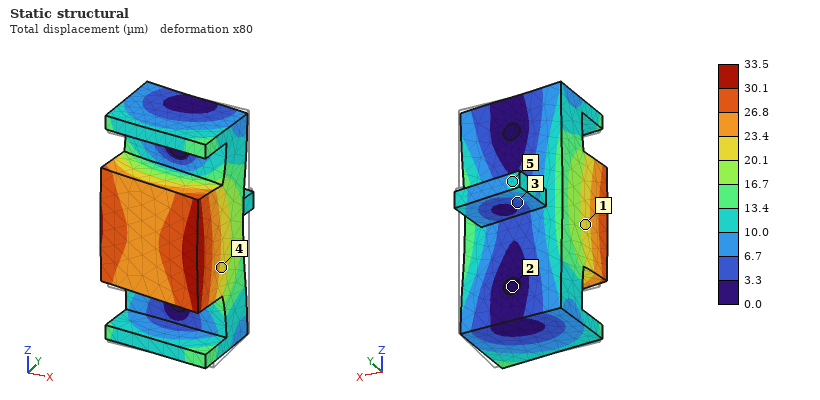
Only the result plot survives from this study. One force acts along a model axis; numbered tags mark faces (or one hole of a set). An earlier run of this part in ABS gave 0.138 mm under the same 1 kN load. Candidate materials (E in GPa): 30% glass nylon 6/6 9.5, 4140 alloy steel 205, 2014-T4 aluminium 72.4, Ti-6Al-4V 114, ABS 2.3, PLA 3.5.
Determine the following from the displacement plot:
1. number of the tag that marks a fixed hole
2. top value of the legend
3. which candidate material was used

2
33.5 µm
30% glass nylon 6/6
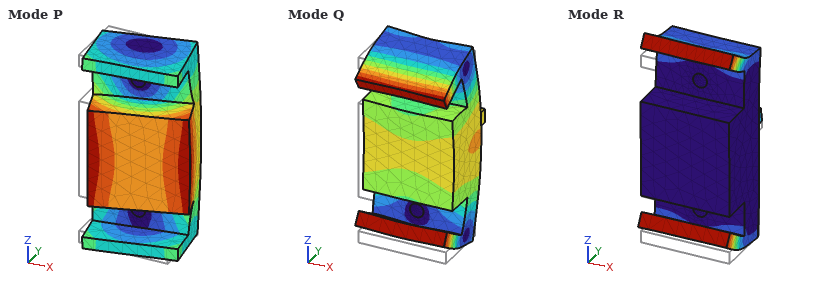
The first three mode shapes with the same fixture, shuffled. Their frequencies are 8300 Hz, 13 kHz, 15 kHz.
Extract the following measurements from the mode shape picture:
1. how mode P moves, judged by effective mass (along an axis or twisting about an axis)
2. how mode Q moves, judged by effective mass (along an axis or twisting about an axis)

along X
along Y
